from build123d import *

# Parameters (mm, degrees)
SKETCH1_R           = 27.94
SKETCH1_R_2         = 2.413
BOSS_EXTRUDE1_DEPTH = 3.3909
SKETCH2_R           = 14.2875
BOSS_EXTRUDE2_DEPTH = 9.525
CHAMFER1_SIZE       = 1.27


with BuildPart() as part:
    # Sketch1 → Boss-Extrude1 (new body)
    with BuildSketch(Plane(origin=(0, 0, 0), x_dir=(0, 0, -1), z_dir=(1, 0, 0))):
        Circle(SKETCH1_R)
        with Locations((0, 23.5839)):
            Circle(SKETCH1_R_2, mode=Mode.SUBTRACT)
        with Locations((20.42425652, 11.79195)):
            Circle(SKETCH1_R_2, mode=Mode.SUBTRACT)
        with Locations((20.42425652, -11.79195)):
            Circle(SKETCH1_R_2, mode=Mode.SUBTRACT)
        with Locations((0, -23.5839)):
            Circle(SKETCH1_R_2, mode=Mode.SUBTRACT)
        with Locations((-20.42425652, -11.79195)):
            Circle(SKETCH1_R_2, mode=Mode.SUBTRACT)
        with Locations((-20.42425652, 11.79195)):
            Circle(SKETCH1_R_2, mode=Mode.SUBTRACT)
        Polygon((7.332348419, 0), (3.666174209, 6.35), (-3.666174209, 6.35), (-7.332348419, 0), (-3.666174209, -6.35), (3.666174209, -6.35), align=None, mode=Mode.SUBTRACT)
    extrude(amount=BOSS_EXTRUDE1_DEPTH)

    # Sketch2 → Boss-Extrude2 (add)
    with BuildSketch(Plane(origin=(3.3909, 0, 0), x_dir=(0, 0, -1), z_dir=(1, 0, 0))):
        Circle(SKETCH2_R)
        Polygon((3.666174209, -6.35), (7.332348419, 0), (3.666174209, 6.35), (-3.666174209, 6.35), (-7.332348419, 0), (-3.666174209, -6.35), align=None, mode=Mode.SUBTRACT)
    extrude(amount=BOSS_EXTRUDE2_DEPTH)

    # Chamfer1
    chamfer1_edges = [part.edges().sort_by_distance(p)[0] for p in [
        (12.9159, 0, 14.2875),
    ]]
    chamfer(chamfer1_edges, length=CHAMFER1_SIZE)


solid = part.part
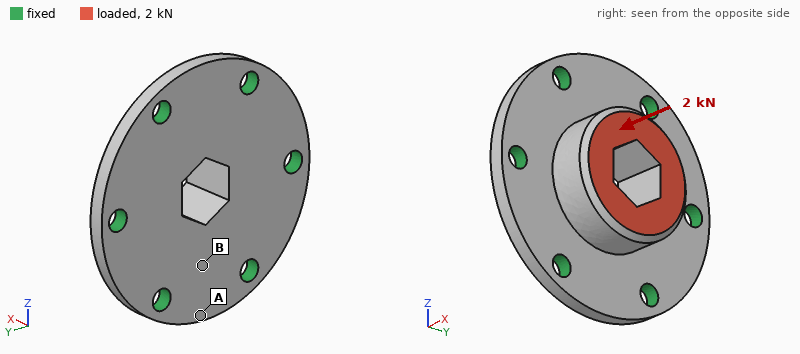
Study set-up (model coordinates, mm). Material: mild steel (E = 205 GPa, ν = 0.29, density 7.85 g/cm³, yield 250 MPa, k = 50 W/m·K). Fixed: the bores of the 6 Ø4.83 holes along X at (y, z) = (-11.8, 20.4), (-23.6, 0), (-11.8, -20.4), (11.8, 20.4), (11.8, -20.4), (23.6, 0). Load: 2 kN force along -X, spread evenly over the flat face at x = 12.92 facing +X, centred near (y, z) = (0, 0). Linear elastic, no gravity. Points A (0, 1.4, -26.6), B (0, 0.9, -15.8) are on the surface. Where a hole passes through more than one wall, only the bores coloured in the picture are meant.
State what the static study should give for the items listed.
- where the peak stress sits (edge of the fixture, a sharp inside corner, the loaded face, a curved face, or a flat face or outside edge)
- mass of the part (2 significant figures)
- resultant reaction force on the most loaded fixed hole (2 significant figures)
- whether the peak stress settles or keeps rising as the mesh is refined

edge of the fixture
96 g
380 N
keeps rising
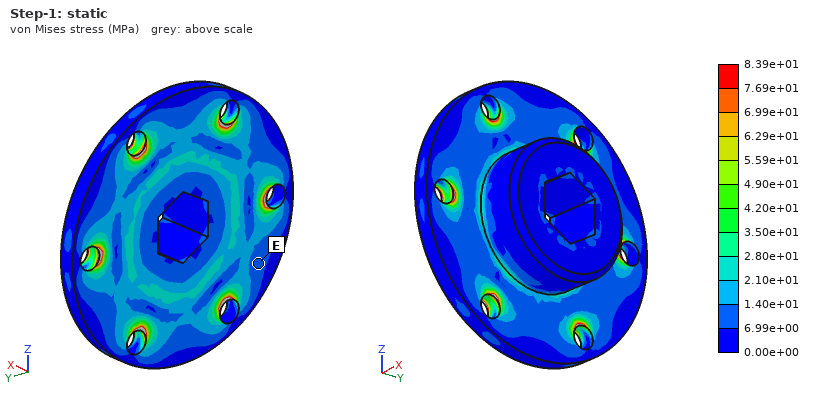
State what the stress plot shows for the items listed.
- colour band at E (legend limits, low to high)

6.99e+00 to 1.40e+01 MPa
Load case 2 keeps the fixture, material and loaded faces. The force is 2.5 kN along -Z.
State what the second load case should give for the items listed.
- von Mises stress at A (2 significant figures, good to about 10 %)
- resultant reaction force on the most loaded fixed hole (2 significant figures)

13 MPa
680 N
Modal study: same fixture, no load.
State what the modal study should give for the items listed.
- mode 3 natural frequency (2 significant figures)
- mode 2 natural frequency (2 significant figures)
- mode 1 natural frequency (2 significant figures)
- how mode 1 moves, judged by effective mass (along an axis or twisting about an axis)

20 kHz
20 kHz
15 kHz
along X
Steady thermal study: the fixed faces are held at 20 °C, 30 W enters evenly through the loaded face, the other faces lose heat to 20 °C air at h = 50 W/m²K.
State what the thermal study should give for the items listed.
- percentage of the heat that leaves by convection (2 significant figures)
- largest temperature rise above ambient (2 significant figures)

11 %
31 K
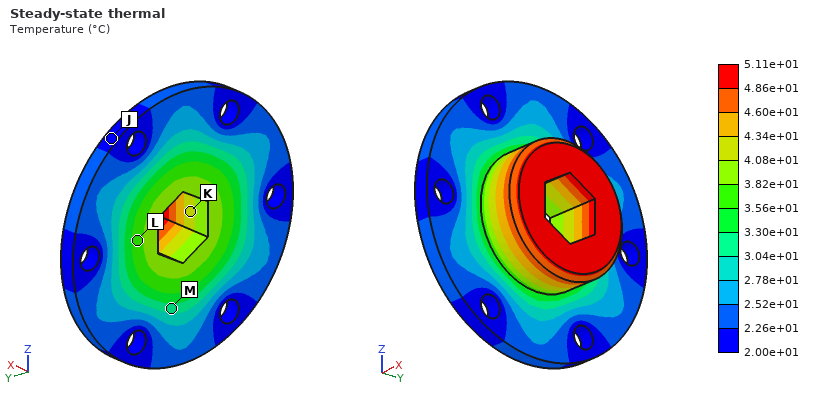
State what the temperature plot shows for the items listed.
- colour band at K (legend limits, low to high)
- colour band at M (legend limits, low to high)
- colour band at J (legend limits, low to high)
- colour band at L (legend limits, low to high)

4.08e+01 to 4.34e+01 °C
3.04e+01 to 3.30e+01 °C
2.00e+01 to 2.26e+01 °C
3.56e+01 to 3.82e+01 °C
